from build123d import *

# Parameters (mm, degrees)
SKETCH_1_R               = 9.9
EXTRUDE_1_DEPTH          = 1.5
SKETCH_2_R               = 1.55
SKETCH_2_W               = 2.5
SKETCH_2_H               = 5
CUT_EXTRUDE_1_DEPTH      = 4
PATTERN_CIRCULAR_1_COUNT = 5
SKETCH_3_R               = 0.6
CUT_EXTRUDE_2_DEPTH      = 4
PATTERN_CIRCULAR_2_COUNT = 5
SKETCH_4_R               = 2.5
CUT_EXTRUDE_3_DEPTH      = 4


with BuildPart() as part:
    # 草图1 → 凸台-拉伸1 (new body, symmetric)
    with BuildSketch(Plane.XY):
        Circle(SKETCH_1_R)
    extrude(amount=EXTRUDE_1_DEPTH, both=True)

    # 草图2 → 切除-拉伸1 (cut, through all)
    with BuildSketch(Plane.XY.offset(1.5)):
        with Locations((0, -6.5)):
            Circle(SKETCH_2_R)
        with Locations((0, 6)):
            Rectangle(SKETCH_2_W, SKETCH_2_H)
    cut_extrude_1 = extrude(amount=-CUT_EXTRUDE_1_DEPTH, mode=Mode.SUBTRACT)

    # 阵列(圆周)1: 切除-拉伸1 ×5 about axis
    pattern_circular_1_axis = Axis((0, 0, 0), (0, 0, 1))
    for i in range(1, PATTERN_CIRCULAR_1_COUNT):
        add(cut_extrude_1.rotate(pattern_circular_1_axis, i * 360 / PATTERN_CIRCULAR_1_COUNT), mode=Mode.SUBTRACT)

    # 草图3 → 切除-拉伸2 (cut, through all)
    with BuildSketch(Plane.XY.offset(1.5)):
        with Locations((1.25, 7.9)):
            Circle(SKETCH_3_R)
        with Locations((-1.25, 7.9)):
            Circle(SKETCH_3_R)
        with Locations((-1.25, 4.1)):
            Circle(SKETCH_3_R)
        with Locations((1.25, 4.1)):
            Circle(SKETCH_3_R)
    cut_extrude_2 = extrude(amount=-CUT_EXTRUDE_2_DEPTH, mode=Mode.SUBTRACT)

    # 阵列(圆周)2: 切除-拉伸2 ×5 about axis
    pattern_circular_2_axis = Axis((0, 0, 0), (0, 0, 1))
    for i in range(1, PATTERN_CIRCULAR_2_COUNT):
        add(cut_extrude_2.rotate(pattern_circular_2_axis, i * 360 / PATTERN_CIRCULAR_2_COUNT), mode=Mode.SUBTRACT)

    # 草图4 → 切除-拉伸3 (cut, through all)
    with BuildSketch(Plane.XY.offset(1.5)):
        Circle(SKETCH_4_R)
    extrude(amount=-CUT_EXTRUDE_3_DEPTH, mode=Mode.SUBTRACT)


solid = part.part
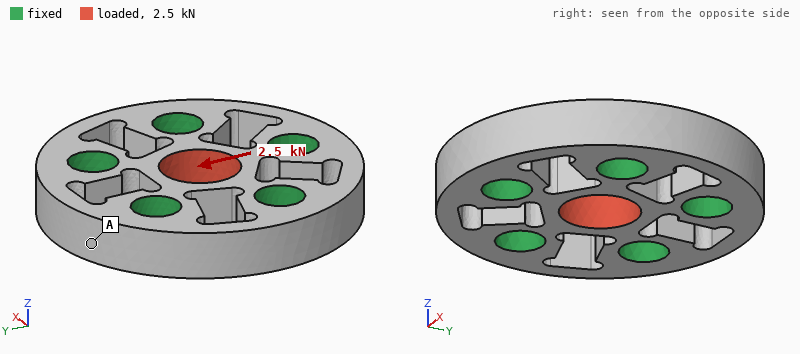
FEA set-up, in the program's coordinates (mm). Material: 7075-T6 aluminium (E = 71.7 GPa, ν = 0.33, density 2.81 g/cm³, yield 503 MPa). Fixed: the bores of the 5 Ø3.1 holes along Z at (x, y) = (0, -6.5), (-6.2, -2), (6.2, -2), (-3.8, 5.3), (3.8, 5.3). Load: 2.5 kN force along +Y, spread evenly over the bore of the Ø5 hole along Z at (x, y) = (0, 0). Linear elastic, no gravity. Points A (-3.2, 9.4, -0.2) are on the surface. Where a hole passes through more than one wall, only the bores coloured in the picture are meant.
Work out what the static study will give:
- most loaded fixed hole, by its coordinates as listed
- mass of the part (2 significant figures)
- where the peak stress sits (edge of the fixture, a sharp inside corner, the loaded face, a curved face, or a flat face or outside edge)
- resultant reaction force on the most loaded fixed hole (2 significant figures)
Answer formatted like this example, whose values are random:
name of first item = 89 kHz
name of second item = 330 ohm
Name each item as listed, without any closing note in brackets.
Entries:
most loaded fixed hole, by its coordinates as listed = (0, -6.5)
mass of the part = 1.5 g
where the peak stress sits = a curved face
resultant reaction force on the most loaded fixed hole = 750 N
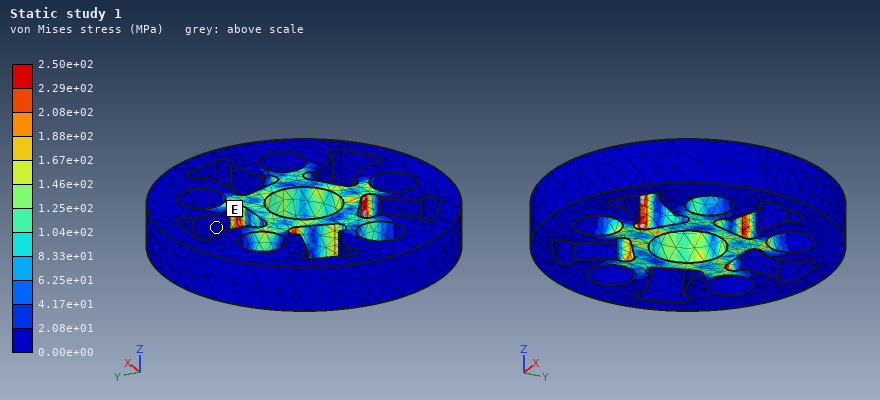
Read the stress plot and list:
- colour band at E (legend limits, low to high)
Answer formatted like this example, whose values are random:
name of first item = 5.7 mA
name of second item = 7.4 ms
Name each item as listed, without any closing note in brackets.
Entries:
colour band at E = 0.00e+00 to 2.08e+01 MPa
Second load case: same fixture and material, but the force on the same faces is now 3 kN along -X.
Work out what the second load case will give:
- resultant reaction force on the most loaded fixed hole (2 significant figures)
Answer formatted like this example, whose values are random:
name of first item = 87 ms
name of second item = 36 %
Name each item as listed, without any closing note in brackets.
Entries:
resultant reaction force on the most loaded fixed hole = 860 N
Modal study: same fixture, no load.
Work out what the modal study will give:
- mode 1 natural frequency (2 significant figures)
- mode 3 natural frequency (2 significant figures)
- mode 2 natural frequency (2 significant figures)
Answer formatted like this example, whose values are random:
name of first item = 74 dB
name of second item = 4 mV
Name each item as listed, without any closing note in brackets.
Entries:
mode 1 natural frequency = 130 kHz
mode 3 natural frequency = 130 kHz
mode 2 natural frequency = 130 kHz
